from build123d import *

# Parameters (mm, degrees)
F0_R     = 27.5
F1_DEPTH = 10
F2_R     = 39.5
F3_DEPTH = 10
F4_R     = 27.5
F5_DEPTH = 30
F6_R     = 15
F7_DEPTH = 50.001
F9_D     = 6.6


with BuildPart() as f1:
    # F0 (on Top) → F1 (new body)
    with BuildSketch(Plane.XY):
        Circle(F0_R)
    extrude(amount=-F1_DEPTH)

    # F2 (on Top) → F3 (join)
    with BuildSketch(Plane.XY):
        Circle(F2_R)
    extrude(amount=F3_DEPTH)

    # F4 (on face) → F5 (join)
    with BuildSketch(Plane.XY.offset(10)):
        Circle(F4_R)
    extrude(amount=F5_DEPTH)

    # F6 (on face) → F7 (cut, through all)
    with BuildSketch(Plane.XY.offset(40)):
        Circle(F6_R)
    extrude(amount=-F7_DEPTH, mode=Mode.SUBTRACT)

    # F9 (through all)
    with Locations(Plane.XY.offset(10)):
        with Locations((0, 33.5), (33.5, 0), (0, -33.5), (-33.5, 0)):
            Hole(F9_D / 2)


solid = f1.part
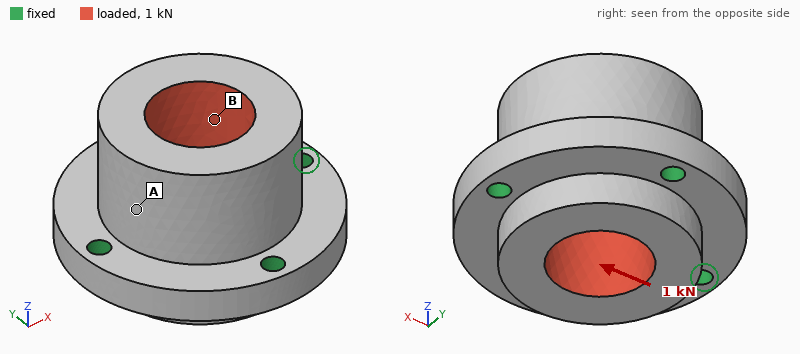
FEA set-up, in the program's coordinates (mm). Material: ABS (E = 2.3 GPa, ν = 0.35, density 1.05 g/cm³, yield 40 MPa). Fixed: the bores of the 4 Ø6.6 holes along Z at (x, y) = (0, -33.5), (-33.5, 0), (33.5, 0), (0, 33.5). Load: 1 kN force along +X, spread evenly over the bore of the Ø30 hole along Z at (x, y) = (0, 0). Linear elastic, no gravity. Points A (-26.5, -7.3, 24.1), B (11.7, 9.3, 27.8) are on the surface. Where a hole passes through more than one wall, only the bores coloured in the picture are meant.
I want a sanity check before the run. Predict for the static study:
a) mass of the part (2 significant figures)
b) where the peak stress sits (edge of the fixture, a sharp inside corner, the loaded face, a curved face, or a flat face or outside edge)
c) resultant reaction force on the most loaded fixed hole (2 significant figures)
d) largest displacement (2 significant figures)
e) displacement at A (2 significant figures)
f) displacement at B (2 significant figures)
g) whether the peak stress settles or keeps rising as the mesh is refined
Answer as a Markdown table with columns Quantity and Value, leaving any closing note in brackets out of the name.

| Quantity | Value |
|---|---|
| mass of the part | 110 g |
| where the peak stress sits | edge of the fixture |
| resultant reaction force on the most loaded fixed hole | 330 N |
| largest displacement | 35 µm |
| displacement at A | 24 µm |
| displacement at B | 25 µm |
| whether the peak stress settles or keeps rising as the mesh is refined | keeps rising |
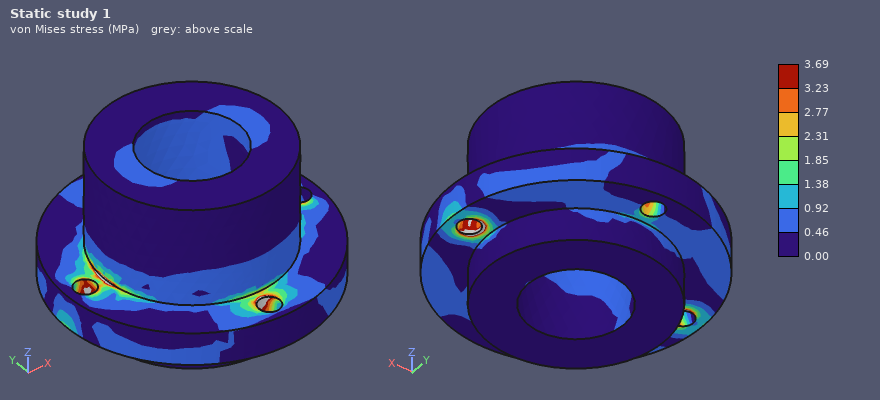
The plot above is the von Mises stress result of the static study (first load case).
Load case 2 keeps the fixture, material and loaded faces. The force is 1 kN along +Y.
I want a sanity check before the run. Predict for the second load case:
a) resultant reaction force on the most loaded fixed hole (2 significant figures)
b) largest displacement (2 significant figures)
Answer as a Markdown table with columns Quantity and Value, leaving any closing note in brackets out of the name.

| Quantity | Value |
|---|---|
| resultant reaction force on the most loaded fixed hole | 330 N |
| largest displacement | 35 µm |
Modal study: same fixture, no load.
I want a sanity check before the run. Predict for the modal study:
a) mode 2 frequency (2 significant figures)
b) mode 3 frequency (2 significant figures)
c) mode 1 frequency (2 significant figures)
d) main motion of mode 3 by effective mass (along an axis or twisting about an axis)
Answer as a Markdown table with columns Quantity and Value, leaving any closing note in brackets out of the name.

| Quantity | Value |
|---|---|
| mode 2 frequency | 3200 Hz |
| mode 3 frequency | 3900 Hz |
| mode 1 frequency | 3200 Hz |
| main motion of mode 3 by effective mass | along Z |
